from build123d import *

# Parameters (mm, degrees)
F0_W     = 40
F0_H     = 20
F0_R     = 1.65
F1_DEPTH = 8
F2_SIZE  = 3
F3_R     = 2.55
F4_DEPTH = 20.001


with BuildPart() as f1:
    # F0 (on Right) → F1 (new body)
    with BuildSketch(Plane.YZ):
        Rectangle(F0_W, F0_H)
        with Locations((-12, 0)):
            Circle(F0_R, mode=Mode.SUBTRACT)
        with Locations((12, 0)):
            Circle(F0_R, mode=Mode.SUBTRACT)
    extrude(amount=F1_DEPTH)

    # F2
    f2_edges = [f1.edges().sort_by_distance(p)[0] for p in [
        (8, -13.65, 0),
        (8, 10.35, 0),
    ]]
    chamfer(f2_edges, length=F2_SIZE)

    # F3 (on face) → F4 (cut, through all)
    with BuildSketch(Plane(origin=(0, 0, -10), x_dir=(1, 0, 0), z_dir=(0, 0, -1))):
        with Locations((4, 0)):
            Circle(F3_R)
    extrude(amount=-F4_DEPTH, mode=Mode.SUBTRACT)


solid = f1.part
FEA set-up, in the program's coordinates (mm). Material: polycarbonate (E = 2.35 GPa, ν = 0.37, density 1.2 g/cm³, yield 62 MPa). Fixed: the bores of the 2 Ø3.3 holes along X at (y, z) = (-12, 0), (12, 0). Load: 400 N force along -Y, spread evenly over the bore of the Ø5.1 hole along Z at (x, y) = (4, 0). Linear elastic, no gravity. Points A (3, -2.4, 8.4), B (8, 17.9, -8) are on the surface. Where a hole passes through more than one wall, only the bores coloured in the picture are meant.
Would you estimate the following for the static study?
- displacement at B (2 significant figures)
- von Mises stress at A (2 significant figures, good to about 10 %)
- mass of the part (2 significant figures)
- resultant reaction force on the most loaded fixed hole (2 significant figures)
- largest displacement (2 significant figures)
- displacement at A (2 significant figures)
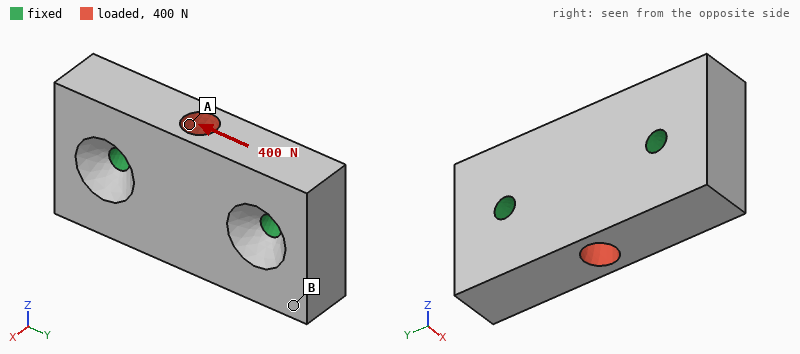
9.6 µm
1.8 MPa
6.8 g
200 N
13 µm
11 µm
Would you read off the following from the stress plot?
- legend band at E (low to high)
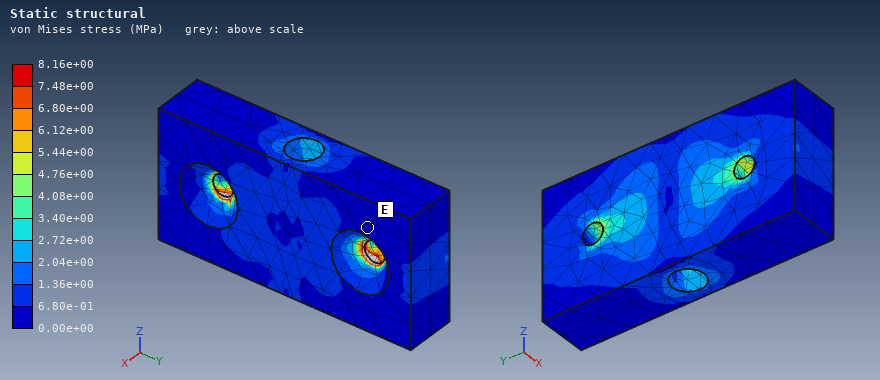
0.00e+00 to 6.80e-01 MPa
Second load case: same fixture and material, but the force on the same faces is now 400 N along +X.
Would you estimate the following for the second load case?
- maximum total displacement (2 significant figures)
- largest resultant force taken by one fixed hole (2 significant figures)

69 µm
210 N
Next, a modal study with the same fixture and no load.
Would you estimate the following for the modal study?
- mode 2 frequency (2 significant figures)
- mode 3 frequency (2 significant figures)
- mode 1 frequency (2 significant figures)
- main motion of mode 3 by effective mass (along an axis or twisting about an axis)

8400 Hz
8900 Hz
5900 Hz
along X
